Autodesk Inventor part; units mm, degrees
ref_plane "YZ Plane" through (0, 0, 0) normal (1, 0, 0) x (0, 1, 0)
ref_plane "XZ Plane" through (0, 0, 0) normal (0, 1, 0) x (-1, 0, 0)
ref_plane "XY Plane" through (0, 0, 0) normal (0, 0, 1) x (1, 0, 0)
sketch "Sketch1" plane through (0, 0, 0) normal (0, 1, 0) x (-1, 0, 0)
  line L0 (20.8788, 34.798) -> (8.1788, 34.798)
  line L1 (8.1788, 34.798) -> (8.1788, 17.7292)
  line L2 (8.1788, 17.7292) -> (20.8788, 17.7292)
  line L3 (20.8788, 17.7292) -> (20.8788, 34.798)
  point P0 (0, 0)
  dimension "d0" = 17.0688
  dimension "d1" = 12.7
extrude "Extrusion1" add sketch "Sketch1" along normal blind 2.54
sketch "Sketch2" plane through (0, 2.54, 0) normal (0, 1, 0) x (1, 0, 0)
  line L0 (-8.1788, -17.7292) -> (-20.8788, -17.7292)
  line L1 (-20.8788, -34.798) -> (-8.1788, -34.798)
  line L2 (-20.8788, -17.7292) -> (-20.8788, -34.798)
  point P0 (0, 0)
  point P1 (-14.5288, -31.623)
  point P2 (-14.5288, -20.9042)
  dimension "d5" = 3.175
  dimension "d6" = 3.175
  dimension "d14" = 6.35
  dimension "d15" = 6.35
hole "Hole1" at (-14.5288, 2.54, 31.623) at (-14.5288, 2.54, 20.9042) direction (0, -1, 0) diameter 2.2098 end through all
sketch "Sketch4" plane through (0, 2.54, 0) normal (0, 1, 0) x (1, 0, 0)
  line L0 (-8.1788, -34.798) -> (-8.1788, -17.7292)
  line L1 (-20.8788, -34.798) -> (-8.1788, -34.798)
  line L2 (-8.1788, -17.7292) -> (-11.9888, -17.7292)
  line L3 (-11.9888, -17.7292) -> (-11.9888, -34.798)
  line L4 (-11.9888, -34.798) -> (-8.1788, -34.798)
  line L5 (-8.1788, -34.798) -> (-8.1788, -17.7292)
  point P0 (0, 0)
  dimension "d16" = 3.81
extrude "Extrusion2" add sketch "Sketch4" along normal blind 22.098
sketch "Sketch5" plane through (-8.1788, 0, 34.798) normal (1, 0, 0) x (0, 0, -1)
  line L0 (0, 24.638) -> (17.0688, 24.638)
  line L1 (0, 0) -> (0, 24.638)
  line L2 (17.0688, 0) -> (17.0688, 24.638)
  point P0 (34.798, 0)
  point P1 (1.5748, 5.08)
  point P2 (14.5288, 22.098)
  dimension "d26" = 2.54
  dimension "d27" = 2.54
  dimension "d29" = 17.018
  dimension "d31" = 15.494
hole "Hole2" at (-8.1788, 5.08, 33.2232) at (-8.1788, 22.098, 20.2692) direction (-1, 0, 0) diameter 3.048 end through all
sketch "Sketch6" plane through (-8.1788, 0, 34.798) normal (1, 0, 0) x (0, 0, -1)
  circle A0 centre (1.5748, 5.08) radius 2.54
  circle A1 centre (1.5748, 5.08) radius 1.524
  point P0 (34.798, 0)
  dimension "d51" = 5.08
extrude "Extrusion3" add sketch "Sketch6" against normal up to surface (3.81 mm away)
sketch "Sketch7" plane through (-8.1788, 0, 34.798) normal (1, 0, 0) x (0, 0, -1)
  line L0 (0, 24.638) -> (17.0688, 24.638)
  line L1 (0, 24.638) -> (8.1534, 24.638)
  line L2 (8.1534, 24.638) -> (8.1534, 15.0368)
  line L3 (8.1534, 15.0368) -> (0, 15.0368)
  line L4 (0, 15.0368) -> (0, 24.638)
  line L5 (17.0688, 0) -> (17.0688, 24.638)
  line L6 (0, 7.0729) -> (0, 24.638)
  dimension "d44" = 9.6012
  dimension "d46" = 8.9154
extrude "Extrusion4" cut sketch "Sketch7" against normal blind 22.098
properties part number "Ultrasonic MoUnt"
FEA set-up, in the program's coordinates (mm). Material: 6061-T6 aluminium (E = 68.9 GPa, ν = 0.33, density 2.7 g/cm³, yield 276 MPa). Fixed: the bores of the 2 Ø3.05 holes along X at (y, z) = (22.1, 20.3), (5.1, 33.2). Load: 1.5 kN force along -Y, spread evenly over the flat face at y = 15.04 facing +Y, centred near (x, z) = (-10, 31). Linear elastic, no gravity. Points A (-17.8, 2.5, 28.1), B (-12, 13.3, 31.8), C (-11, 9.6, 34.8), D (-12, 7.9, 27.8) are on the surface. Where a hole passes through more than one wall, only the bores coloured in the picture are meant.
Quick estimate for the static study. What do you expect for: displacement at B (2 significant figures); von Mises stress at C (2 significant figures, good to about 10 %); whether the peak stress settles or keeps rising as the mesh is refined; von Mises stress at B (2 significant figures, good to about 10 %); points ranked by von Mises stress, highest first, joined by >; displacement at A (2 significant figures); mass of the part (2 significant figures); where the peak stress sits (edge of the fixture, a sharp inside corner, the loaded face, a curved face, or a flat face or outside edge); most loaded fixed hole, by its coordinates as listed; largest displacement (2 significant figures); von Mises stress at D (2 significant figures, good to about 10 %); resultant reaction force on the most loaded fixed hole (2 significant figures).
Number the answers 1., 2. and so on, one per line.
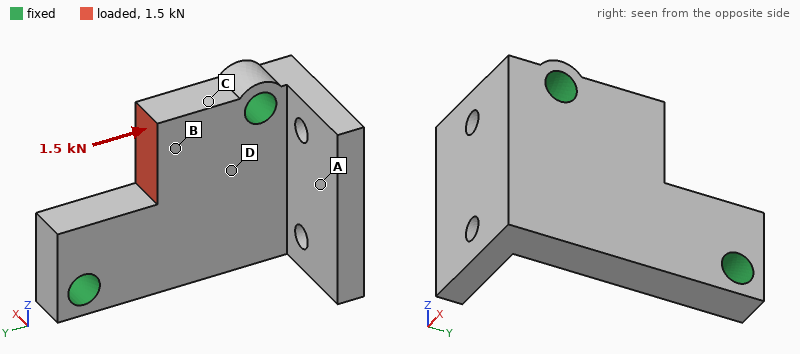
1. 5.5 µm
2. 61 MPa
3. keeps rising
4. 48 MPa
5. C > B > D > A
6. 1.6 µm
7. 4.4 g
8. edge of the fixture
9. (5.1, 33.2)
10. 6.9 µm
11. 16 MPa
12. 1.1 kN
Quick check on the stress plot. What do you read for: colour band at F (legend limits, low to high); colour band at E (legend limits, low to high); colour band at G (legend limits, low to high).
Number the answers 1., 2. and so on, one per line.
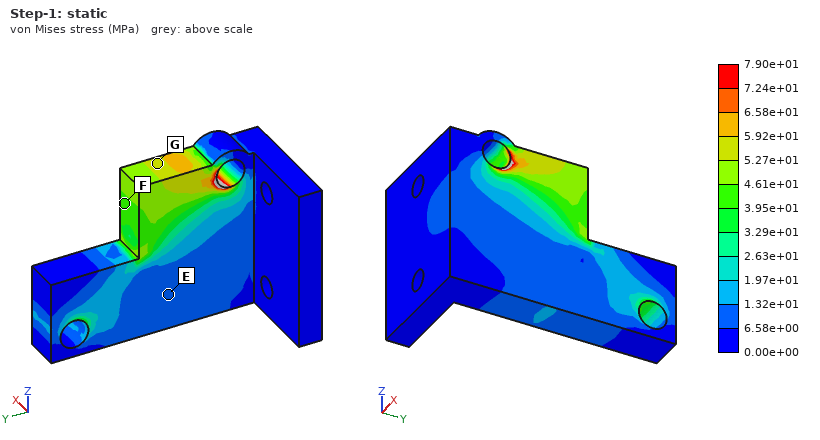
1. 3.95e+01 to 4.61e+01 MPa
2. 6.58e+00 to 1.32e+01 MPa
3. 5.27e+01 to 5.92e+01 MPa
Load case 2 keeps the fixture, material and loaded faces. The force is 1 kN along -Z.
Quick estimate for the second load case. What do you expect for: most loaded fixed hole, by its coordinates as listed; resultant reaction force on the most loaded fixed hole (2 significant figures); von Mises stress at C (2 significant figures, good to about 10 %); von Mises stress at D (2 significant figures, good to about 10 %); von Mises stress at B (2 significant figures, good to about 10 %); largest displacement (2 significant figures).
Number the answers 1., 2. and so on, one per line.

1. (5.1, 33.2)
2. 800 N
3. 47 MPa
4. 29 MPa
5. 42 MPa
6. 18 µm
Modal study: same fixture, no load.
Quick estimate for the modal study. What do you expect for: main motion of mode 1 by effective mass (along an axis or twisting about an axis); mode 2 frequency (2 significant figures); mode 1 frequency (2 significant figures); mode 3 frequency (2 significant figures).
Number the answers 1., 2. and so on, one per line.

1. along X
2. 16 kHz
3. 12 kHz
4. 27 kHz
